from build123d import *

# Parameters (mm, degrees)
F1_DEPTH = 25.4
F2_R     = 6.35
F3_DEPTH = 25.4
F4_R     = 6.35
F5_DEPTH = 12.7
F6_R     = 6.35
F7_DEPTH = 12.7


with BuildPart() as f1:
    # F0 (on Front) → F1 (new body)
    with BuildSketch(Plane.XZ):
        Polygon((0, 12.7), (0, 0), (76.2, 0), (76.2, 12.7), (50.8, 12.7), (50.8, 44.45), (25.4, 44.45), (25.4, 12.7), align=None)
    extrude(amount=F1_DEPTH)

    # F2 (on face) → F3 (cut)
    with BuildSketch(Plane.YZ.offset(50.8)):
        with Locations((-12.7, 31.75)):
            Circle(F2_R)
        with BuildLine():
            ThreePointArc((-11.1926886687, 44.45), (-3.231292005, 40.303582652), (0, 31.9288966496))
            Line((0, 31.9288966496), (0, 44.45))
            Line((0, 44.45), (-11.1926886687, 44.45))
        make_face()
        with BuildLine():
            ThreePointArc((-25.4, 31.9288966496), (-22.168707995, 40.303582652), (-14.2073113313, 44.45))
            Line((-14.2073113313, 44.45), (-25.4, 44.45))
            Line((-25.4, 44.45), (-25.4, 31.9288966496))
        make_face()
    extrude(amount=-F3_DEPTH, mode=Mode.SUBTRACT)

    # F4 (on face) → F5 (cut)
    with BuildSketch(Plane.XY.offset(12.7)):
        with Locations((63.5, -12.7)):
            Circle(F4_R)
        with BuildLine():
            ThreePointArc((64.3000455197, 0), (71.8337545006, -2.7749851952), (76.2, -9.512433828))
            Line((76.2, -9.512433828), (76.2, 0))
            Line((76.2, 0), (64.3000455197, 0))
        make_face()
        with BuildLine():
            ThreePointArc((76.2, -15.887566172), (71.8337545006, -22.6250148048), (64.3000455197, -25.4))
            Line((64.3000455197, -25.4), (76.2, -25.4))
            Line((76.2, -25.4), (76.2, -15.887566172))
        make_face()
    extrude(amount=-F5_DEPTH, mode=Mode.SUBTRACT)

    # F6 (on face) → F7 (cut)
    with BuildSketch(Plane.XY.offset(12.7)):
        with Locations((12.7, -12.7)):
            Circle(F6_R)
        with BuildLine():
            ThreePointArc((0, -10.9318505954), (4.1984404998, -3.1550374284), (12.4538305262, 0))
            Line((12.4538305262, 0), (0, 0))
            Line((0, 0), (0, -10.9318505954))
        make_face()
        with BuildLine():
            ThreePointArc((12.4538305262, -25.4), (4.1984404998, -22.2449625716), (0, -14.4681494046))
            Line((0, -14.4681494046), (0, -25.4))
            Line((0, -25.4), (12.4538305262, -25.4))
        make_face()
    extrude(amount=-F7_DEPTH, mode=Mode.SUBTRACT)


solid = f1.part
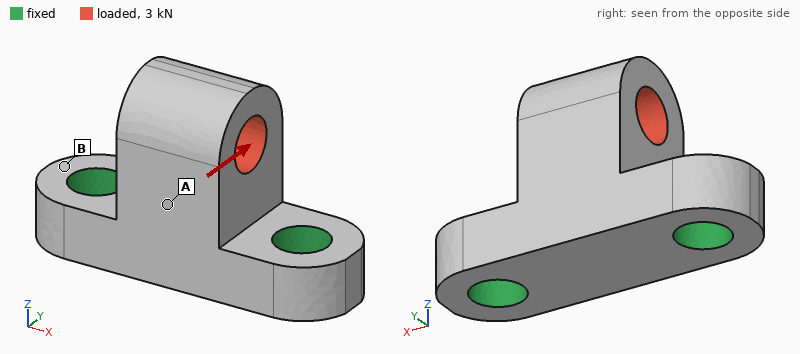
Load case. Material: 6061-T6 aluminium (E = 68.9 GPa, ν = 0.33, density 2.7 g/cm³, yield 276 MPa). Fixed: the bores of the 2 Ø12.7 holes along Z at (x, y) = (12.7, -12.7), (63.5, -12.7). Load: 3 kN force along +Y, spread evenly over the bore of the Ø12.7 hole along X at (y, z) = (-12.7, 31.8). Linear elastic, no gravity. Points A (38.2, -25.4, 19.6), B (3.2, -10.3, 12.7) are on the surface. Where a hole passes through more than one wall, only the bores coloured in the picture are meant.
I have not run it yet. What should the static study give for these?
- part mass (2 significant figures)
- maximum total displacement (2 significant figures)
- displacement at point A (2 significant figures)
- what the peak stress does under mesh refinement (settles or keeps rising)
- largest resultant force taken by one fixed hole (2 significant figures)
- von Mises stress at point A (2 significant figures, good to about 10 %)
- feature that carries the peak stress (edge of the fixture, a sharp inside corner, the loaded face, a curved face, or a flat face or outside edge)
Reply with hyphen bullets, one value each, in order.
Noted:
- 95 g
- 66 µm
- 29 µm
- keeps rising
- 1.5 kN
- 14 MPa
- edge of the fixture
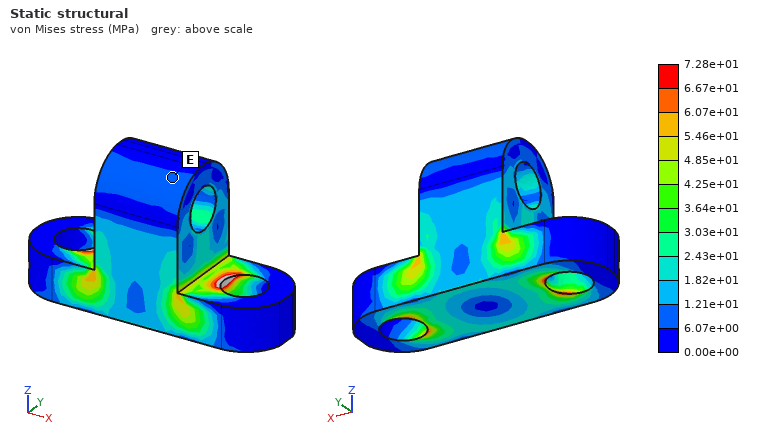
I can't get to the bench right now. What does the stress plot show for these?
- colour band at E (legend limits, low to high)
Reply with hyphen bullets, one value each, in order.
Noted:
- 6.07e+00 to 1.21e+01 MPa
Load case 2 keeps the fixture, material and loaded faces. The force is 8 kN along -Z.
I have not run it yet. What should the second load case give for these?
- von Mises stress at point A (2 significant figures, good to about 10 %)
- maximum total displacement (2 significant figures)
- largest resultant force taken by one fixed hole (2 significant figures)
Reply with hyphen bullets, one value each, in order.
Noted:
- 11 MPa
- 18 µm
- 4.2 kN
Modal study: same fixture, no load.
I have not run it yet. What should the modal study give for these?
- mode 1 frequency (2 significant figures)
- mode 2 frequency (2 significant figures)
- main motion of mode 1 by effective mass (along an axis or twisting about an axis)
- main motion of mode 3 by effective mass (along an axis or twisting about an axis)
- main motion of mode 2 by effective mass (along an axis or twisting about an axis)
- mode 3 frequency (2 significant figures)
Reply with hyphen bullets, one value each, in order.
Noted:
- 6900 Hz
- 12 kHz
- along Y
- along Z
- along X
- 17 kHz
